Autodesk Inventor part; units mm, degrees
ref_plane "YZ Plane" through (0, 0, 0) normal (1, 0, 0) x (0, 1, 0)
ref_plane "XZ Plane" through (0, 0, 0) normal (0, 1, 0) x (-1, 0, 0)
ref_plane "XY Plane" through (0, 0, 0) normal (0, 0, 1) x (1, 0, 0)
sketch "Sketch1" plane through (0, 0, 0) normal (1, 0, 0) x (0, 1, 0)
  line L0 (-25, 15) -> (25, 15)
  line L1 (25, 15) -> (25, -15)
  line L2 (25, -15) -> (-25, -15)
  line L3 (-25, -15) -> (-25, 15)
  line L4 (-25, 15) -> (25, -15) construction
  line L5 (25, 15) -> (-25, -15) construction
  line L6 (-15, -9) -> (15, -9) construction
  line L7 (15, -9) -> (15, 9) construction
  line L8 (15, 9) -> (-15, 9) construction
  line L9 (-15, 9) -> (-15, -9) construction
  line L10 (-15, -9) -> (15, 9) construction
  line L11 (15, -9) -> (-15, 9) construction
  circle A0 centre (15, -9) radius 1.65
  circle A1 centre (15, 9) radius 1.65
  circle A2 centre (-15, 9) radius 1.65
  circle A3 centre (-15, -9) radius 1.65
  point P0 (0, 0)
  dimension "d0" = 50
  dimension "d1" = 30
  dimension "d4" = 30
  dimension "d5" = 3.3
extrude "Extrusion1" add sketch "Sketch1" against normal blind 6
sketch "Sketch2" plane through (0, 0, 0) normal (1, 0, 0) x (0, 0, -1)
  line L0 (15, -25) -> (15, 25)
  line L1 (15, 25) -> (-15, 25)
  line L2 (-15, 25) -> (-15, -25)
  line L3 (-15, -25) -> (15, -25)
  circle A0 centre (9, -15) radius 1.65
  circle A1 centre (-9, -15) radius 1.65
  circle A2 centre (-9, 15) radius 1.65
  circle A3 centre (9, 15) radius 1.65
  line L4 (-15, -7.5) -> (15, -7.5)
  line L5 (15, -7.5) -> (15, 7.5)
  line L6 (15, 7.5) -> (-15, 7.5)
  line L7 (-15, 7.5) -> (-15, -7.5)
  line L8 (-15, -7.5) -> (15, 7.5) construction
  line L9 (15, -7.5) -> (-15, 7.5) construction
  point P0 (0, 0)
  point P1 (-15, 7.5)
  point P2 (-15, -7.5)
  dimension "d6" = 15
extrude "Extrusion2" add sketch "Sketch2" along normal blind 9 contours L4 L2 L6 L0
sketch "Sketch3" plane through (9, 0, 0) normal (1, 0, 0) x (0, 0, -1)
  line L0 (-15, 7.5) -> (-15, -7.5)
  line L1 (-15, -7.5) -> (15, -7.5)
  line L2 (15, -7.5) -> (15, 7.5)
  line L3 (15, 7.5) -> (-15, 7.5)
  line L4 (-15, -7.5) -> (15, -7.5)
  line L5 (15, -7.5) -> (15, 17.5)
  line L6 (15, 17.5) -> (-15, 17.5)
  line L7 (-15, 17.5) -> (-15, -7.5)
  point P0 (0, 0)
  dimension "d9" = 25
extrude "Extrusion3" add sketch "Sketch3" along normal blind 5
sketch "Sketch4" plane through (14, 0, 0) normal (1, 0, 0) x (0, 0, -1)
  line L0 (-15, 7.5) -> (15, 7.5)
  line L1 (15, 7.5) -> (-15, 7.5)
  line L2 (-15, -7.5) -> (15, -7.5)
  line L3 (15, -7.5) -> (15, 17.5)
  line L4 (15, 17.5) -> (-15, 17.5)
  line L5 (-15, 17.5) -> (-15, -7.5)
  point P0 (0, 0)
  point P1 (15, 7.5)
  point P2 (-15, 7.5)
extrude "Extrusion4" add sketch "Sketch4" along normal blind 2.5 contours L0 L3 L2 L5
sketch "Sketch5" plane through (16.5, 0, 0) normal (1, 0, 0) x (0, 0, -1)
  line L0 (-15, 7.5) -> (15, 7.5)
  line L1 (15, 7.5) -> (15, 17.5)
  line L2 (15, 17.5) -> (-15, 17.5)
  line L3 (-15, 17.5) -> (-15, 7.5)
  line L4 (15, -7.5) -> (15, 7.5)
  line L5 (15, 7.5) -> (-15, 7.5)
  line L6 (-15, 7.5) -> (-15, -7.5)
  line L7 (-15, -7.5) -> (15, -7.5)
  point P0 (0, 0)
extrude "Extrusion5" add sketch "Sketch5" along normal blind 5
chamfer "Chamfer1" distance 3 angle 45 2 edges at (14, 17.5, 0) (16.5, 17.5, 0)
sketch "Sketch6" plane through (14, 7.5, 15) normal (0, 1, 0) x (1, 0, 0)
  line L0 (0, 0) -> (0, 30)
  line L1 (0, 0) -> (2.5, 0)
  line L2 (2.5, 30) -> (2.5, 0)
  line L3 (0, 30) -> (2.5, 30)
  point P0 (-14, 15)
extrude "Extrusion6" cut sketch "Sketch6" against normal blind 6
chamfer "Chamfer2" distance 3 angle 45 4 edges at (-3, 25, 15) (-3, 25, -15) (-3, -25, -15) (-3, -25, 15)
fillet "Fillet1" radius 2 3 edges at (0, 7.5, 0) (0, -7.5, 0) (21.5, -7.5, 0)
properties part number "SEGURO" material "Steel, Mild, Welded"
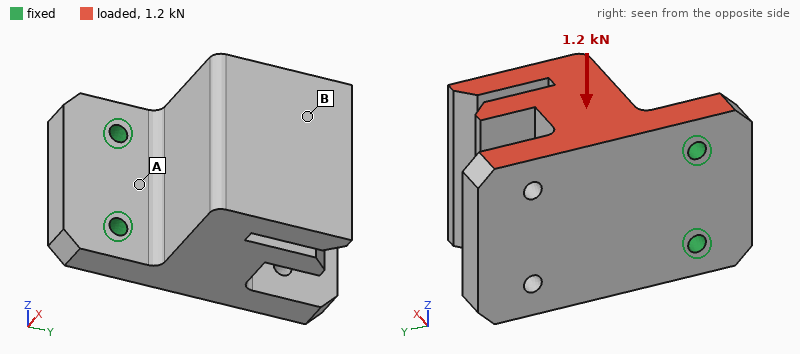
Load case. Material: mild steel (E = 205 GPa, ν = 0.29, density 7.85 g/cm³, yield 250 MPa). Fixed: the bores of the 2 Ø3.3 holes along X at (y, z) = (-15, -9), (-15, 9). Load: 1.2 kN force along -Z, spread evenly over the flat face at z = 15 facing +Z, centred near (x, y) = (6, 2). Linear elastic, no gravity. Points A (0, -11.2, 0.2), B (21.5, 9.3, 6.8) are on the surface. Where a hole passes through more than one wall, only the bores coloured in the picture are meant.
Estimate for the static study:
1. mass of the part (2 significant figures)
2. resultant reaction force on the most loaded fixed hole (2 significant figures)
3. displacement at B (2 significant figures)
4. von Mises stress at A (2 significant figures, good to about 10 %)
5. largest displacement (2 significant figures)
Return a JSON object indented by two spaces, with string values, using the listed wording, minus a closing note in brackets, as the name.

{
  "mass of the part": "160 g",
  "resultant reaction force on the most loaded fixed hole": "1.3 kN",
  "displacement at B": "7.0 µm",
  "von Mises stress at A": "23 MPa",
  "largest displacement": "8.1 µm"
}
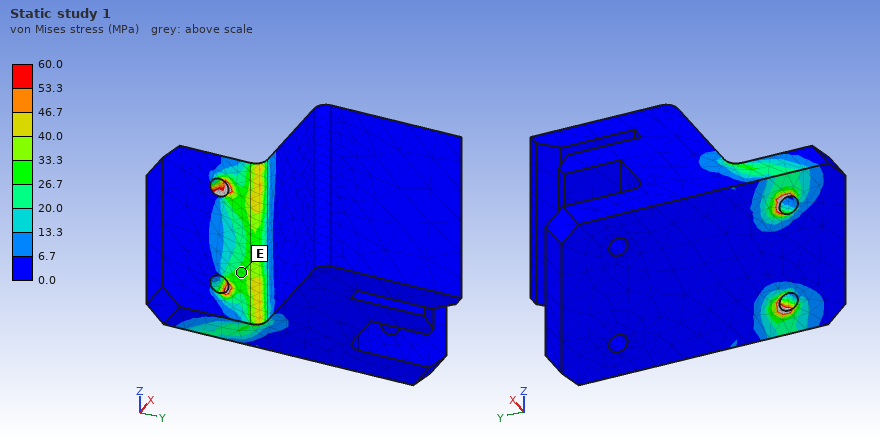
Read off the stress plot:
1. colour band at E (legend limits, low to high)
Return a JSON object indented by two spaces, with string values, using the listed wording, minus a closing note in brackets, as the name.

{
  "colour band at E": "26.7 to 33.3 MPa"
}
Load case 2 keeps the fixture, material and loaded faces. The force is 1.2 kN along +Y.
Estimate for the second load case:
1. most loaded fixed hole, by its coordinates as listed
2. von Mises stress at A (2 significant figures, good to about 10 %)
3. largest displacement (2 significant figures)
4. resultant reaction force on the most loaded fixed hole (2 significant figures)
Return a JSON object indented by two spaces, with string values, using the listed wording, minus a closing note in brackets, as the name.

{
  "most loaded fixed hole, by its coordinates as listed": "(-15, 9)",
  "von Mises stress at A": "44 MPa",
  "largest displacement": "40 µm",
  "resultant reaction force on the most loaded fixed hole": "1.5 kN"
}
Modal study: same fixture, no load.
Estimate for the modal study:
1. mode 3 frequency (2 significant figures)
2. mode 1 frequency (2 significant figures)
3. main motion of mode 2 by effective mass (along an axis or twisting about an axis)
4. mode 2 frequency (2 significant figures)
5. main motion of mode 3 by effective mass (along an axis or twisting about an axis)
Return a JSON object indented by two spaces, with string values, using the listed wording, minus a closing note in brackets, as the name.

{
  "mode 3 frequency": "8900 Hz",
  "mode 1 frequency": "2000 Hz",
  "main motion of mode 2 by effective mass": "along Z",
  "mode 2 frequency": "5900 Hz",
  "main motion of mode 3 by effective mass": "along Z"
}
